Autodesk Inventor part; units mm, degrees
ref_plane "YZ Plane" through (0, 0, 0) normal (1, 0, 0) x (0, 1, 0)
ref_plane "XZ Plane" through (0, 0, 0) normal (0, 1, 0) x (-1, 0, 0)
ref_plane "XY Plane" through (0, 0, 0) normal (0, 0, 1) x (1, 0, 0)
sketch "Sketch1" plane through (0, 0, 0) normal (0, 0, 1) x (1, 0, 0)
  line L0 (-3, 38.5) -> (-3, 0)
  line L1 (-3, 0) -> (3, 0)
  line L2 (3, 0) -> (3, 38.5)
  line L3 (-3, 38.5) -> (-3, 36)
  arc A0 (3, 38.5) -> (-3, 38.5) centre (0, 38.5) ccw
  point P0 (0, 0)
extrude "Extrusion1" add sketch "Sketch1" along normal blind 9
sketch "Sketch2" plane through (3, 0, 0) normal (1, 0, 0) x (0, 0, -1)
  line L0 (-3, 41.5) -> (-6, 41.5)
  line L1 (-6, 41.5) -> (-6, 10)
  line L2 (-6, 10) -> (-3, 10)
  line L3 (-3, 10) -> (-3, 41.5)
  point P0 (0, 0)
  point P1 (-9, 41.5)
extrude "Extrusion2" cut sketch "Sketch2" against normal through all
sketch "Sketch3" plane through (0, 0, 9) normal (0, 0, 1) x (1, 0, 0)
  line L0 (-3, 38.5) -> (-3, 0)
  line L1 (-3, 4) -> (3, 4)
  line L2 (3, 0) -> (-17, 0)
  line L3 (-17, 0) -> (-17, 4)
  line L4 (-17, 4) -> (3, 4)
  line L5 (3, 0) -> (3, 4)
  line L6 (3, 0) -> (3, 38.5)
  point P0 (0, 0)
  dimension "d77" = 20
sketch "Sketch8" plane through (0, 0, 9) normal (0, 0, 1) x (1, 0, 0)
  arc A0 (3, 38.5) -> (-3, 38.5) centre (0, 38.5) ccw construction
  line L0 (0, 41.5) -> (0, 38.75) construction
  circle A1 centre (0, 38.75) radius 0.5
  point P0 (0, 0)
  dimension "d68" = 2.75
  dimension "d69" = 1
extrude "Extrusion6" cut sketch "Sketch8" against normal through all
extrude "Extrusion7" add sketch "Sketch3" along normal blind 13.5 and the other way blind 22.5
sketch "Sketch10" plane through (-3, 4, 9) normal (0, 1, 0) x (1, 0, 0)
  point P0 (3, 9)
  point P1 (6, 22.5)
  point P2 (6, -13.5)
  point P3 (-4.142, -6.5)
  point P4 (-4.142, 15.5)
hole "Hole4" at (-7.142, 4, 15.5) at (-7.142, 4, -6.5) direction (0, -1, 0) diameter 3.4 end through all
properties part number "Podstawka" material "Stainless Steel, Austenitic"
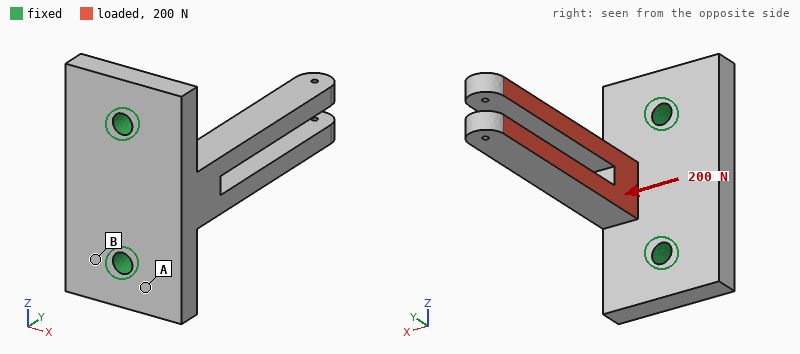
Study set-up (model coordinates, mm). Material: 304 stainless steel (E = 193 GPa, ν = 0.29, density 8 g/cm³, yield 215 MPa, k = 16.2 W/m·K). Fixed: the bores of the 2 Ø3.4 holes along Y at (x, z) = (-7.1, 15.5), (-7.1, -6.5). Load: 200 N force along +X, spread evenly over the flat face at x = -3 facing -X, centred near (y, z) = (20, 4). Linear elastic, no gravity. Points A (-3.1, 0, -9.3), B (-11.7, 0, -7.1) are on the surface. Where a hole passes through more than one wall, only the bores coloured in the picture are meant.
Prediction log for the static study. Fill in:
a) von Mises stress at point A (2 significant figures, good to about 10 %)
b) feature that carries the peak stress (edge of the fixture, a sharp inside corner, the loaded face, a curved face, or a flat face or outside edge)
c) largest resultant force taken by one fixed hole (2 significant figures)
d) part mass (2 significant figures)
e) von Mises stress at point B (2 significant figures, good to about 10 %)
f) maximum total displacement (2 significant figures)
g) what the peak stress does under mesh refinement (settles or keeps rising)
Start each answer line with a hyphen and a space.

- 24 MPa
- edge of the fixture
- 100 N
- 34 g
- 8.1 MPa
- 89 µm
- keeps rising
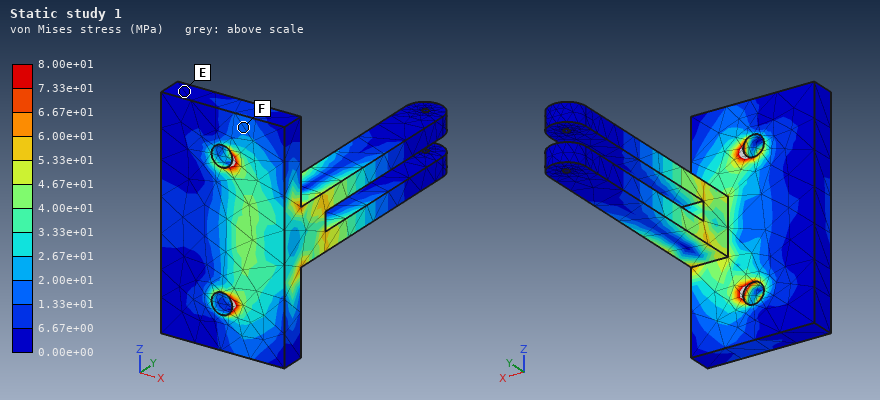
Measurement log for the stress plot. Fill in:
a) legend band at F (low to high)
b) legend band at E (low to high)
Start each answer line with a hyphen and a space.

- 1.33e+01 to 2.00e+01 MPa
- 0.00e+00 to 6.67e+00 MPa
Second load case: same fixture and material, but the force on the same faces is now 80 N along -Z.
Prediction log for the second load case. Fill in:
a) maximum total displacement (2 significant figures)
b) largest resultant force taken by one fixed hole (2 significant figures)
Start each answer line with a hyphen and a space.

- 55 µm
- 92 N
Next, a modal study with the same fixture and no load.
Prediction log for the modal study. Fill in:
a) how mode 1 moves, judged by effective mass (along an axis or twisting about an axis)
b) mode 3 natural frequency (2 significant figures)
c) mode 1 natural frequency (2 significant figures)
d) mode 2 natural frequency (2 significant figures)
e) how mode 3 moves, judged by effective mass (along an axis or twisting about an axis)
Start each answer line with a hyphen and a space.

- along Z
- 2700 Hz
- 2100 Hz
- 2300 Hz
- along X
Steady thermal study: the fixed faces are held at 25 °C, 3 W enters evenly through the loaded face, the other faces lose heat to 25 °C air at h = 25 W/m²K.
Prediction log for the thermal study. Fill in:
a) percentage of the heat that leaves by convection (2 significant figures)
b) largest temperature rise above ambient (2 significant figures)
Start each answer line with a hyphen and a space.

- 42 %
- 51 K
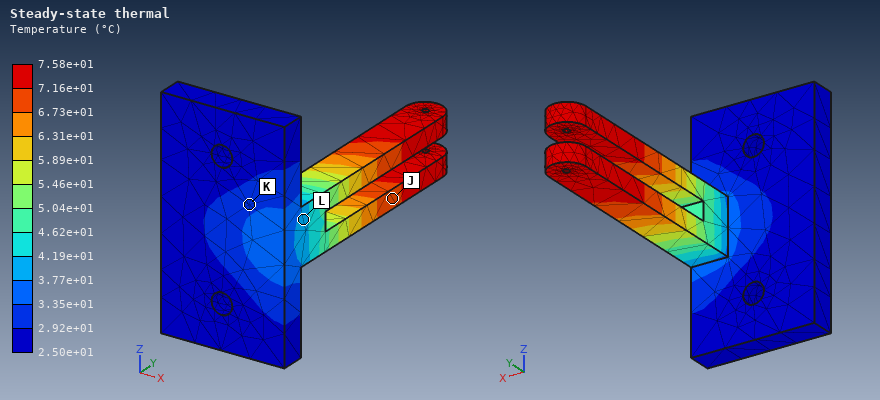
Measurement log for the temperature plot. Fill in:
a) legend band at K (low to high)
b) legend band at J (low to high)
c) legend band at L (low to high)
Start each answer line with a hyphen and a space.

- 2.92e+01 to 3.35e+01 °C
- 6.73e+01 to 7.16e+01 °C
- 3.77e+01 to 4.19e+01 °C
